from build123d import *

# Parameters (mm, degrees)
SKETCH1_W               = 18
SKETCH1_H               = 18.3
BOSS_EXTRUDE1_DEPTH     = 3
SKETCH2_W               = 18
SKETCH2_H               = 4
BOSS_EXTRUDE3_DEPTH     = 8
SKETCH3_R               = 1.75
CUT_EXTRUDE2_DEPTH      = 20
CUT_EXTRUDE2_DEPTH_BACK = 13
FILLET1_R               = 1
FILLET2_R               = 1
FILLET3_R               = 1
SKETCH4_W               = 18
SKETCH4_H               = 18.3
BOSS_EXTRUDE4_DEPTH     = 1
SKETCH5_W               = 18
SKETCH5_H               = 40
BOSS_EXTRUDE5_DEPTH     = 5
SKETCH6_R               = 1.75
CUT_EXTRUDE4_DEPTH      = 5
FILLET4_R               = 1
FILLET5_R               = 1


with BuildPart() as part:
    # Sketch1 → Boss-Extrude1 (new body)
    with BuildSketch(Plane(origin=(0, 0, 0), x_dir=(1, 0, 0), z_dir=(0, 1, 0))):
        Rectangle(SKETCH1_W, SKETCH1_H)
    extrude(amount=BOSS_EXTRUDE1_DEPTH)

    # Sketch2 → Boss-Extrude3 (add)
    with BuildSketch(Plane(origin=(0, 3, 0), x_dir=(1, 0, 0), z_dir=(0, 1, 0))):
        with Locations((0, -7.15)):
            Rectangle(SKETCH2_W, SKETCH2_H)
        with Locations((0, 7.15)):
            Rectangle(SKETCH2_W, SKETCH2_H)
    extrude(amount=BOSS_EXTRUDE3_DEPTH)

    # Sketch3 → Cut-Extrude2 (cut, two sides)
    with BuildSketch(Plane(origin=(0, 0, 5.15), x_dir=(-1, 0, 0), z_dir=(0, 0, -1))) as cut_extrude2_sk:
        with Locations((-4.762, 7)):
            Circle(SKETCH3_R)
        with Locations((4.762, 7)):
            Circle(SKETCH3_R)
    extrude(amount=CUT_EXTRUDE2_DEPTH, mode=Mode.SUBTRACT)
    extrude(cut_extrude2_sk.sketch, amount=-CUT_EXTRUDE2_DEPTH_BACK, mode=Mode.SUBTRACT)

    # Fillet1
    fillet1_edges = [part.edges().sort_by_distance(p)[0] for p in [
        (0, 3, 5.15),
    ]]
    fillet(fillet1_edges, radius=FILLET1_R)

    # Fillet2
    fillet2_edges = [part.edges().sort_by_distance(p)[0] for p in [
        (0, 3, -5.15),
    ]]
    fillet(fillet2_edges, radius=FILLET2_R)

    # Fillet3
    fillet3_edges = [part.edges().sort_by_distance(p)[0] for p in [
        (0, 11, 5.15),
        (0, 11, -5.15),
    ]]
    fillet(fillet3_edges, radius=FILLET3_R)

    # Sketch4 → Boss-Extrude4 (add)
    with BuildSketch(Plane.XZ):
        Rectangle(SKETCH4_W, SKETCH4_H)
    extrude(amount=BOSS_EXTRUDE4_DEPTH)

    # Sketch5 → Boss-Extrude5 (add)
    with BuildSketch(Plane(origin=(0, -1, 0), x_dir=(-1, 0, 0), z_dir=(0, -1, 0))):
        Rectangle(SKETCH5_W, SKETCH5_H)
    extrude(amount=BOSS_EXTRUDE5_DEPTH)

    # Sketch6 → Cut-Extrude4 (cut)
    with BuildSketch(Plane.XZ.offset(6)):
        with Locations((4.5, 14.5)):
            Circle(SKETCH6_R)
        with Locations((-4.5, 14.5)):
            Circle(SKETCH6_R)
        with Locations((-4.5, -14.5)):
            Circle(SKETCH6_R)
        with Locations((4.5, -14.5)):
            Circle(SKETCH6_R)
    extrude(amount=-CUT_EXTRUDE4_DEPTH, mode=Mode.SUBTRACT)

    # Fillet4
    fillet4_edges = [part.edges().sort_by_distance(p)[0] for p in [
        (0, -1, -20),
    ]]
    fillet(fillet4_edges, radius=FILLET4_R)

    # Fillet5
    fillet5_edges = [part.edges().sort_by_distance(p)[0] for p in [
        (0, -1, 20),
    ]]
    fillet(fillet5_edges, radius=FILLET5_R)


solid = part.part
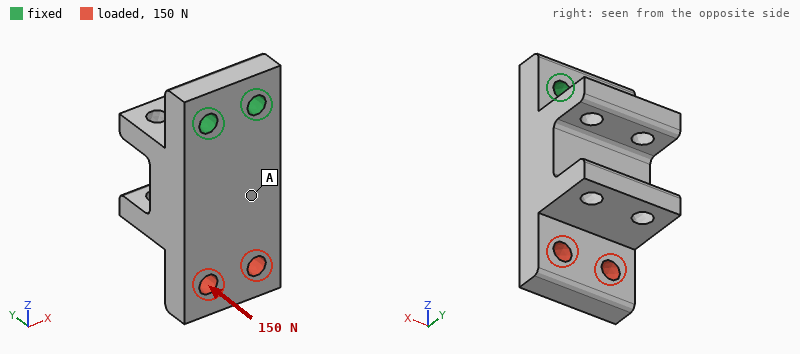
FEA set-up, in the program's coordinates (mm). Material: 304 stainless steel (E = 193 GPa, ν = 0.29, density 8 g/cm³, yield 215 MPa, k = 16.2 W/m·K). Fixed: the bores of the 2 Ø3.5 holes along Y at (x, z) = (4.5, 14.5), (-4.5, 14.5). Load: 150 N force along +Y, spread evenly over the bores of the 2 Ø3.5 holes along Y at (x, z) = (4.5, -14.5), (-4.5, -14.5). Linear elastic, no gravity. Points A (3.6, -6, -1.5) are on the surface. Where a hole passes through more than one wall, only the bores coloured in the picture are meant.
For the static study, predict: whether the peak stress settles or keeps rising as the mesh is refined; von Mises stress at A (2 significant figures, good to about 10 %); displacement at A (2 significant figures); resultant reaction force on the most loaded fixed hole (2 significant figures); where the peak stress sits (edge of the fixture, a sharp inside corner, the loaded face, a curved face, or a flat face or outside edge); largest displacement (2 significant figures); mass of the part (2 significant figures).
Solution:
keeps rising
8.4 MPa
9.2 µm
75 N
edge of the fixture
26 µm
46 g
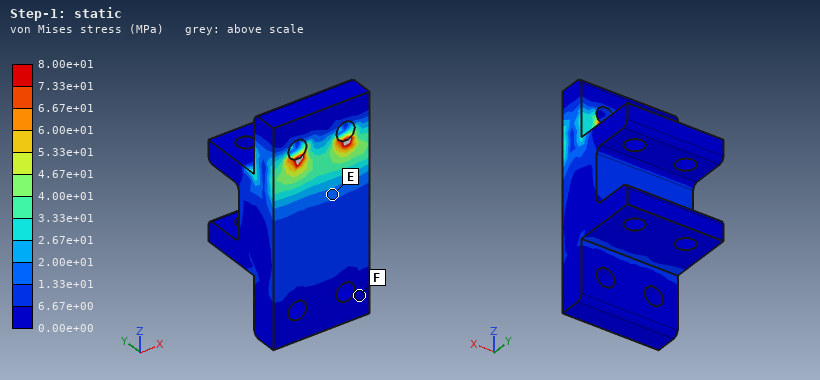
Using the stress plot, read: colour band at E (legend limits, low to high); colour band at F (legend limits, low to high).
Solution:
1.33e+01 to 2.00e+01 MPa
0.00e+00 to 6.67e+00 MPa
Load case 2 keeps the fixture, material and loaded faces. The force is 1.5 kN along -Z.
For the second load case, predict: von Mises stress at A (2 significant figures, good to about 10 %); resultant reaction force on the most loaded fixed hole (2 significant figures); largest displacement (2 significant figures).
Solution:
21 MPa
760 N
5.6 µm
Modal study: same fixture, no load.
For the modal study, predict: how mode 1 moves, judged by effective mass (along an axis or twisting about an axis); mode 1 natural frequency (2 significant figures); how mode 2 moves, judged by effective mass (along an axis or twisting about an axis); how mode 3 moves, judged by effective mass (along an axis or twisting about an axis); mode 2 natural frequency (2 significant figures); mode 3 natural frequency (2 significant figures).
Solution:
along Y
3500 Hz
along X
twisting about Z
9100 Hz
12 kHz
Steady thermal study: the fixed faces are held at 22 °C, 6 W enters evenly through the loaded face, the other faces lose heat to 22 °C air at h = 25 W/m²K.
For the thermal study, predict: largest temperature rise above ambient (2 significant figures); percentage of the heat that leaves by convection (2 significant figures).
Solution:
74 K
37 %
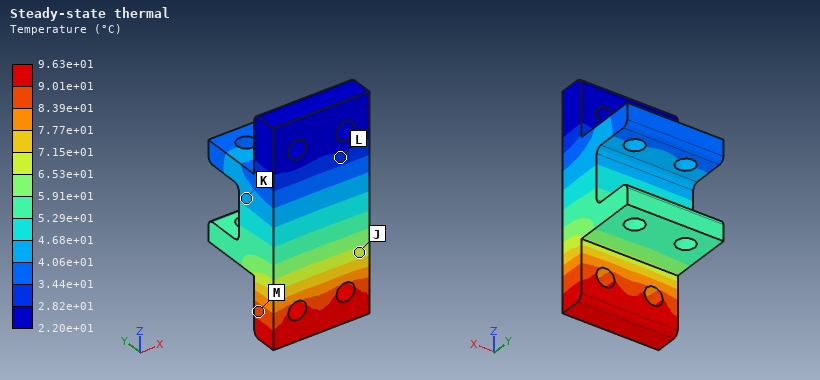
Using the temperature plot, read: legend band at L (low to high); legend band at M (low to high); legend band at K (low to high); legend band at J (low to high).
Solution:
2.82e+01 to 3.44e+01 °C
8.39e+01 to 9.01e+01 °C
4.06e+01 to 4.68e+01 °C
6.53e+01 to 7.15e+01 °C
